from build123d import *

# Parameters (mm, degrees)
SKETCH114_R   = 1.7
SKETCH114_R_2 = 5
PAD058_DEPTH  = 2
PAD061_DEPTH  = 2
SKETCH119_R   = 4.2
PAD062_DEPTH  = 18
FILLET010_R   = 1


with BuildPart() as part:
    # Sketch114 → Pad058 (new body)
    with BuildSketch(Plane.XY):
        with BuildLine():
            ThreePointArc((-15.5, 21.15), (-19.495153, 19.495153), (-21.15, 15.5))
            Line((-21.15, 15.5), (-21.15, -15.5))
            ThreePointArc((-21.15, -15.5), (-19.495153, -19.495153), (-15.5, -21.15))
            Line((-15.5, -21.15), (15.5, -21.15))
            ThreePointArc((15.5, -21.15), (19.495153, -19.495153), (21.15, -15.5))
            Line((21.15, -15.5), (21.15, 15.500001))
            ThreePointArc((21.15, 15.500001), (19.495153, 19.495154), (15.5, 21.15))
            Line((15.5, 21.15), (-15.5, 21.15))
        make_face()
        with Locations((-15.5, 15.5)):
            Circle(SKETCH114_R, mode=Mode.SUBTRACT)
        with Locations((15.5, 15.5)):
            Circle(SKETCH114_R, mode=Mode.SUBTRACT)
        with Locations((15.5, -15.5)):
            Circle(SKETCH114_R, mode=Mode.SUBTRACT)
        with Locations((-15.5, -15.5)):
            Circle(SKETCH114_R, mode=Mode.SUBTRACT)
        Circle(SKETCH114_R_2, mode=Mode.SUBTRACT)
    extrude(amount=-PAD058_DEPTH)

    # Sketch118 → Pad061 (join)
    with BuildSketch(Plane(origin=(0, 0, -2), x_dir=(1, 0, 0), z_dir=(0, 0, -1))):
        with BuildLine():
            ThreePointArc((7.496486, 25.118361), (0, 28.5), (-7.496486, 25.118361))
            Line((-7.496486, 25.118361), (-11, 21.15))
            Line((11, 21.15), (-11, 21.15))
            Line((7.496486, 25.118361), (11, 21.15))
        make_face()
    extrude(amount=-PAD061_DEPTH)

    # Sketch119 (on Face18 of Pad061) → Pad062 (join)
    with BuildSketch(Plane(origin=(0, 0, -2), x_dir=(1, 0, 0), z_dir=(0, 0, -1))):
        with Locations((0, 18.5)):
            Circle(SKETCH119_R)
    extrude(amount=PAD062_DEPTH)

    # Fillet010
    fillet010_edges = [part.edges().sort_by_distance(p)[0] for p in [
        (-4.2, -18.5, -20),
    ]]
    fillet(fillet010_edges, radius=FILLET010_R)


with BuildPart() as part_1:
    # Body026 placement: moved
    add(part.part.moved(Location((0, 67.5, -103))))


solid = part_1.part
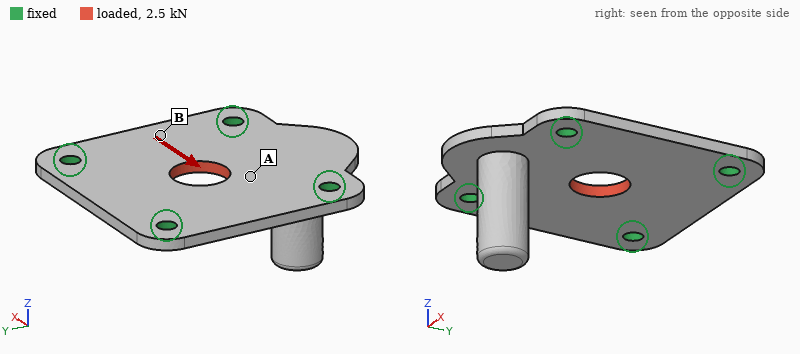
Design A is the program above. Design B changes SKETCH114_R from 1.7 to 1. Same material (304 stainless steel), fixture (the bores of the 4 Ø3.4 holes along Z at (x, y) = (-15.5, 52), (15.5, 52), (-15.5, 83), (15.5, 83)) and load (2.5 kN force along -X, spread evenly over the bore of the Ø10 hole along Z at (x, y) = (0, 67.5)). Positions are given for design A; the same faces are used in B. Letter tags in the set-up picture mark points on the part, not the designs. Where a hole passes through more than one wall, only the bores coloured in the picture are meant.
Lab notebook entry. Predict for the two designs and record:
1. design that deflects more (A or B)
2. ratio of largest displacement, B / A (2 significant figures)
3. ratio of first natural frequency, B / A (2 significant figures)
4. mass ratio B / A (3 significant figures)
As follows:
B
1.1
0.95
1.01
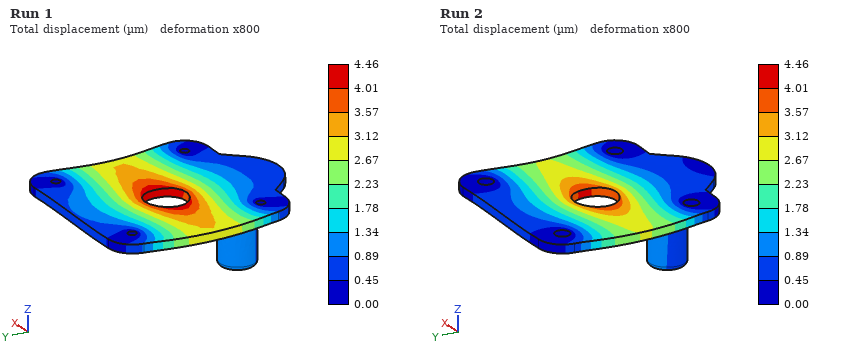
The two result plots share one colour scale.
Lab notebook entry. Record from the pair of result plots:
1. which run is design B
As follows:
Run 1
